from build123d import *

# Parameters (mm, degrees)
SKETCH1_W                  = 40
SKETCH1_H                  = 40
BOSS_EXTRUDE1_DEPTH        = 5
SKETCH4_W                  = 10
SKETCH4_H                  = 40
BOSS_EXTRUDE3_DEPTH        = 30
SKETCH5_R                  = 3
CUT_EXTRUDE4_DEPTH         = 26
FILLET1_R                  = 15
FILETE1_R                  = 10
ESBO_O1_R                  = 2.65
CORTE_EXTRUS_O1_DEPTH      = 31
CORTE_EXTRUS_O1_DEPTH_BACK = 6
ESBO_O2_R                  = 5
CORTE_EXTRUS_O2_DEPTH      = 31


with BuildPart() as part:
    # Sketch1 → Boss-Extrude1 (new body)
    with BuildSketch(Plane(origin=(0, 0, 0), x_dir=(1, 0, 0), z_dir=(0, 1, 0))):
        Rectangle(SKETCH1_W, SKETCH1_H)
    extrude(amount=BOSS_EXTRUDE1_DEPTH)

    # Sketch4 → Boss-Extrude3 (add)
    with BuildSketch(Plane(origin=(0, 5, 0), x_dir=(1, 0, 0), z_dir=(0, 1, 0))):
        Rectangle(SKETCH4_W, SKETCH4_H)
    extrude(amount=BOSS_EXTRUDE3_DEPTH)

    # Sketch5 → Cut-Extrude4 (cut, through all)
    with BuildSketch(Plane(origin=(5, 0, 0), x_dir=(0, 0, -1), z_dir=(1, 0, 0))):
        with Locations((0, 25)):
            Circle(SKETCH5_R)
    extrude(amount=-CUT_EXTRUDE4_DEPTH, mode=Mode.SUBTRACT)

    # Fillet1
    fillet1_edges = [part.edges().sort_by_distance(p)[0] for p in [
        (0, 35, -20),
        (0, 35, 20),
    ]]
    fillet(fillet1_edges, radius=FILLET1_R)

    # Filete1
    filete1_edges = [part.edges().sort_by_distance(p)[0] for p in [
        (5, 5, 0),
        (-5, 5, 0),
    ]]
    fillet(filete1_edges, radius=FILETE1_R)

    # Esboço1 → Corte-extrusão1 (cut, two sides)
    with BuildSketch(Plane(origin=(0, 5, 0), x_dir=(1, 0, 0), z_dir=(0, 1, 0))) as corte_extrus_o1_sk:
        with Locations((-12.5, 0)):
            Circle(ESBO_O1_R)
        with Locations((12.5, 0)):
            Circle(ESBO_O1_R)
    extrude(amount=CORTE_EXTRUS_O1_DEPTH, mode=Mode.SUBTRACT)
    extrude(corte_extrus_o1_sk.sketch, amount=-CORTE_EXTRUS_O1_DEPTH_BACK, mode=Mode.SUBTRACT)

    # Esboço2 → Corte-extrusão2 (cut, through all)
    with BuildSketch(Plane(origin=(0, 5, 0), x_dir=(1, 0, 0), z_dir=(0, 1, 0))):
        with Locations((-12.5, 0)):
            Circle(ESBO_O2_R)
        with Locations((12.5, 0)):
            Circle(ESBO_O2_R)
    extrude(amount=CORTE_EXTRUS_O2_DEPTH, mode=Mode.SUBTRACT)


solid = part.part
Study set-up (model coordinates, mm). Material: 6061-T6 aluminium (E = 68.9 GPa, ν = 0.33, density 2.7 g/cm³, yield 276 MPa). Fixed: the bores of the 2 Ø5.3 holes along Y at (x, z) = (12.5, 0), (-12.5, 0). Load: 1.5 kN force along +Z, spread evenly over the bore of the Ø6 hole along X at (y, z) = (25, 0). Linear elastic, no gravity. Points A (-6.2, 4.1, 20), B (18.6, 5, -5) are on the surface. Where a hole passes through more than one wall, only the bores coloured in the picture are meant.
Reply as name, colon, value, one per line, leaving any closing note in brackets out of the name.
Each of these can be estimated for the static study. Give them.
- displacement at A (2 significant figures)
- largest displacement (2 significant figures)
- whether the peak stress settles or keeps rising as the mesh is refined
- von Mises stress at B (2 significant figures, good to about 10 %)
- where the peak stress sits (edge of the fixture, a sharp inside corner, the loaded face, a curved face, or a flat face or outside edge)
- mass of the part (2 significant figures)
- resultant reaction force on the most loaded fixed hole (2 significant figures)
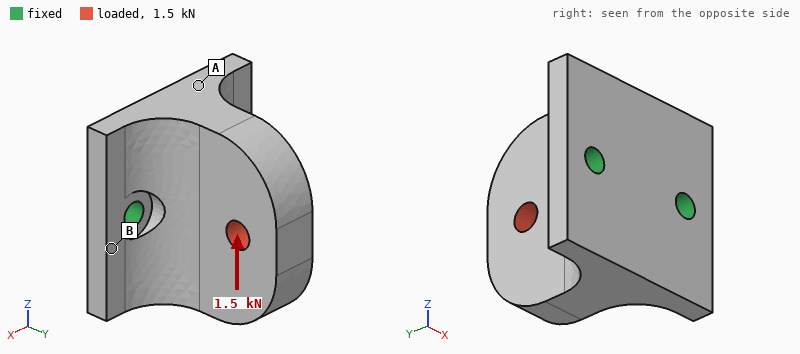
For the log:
displacement at A: 56 µm
largest displacement: 97 µm
whether the peak stress settles or keeps rising as the mesh is refined: keeps rising
von Mises stress at B: 45 MPa
where the peak stress sits: edge of the fixture
mass of the part: 54 g
resultant reaction force on the most loaded fixed hole: 750 N
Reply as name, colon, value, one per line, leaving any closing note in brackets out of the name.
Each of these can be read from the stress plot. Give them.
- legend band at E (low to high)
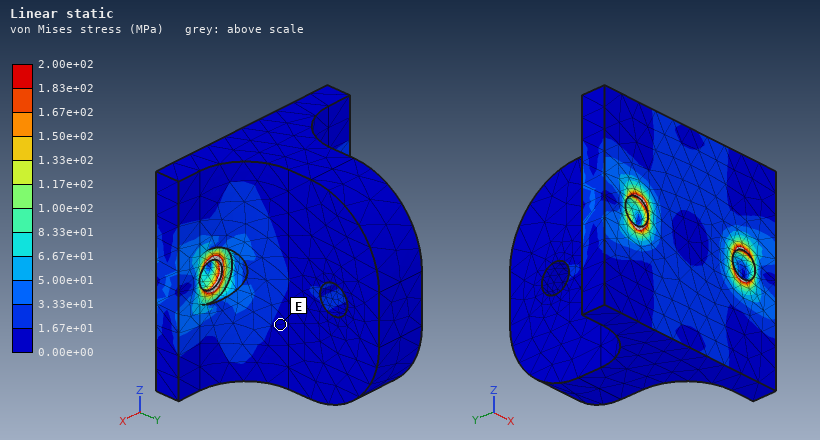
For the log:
legend band at E: 0.00e+00 to 1.67e+01 MPa
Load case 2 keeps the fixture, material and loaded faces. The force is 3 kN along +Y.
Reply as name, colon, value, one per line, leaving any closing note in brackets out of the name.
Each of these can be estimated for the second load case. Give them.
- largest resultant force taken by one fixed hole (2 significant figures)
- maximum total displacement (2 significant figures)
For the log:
largest resultant force taken by one fixed hole: 1.6 kN
maximum total displacement: 12 µm
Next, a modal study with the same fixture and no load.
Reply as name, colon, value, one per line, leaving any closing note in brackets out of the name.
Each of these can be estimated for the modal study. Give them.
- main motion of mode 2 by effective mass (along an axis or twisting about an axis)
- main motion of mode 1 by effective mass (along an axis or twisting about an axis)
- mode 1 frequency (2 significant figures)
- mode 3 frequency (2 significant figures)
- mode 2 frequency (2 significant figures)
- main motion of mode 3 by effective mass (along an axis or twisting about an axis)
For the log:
main motion of mode 2 by effective mass: along X
main motion of mode 1 by effective mass: along Z
mode 1 frequency: 4300 Hz
mode 3 frequency: 15 kHz
mode 2 frequency: 8800 Hz
main motion of mode 3 by effective mass: along Y
